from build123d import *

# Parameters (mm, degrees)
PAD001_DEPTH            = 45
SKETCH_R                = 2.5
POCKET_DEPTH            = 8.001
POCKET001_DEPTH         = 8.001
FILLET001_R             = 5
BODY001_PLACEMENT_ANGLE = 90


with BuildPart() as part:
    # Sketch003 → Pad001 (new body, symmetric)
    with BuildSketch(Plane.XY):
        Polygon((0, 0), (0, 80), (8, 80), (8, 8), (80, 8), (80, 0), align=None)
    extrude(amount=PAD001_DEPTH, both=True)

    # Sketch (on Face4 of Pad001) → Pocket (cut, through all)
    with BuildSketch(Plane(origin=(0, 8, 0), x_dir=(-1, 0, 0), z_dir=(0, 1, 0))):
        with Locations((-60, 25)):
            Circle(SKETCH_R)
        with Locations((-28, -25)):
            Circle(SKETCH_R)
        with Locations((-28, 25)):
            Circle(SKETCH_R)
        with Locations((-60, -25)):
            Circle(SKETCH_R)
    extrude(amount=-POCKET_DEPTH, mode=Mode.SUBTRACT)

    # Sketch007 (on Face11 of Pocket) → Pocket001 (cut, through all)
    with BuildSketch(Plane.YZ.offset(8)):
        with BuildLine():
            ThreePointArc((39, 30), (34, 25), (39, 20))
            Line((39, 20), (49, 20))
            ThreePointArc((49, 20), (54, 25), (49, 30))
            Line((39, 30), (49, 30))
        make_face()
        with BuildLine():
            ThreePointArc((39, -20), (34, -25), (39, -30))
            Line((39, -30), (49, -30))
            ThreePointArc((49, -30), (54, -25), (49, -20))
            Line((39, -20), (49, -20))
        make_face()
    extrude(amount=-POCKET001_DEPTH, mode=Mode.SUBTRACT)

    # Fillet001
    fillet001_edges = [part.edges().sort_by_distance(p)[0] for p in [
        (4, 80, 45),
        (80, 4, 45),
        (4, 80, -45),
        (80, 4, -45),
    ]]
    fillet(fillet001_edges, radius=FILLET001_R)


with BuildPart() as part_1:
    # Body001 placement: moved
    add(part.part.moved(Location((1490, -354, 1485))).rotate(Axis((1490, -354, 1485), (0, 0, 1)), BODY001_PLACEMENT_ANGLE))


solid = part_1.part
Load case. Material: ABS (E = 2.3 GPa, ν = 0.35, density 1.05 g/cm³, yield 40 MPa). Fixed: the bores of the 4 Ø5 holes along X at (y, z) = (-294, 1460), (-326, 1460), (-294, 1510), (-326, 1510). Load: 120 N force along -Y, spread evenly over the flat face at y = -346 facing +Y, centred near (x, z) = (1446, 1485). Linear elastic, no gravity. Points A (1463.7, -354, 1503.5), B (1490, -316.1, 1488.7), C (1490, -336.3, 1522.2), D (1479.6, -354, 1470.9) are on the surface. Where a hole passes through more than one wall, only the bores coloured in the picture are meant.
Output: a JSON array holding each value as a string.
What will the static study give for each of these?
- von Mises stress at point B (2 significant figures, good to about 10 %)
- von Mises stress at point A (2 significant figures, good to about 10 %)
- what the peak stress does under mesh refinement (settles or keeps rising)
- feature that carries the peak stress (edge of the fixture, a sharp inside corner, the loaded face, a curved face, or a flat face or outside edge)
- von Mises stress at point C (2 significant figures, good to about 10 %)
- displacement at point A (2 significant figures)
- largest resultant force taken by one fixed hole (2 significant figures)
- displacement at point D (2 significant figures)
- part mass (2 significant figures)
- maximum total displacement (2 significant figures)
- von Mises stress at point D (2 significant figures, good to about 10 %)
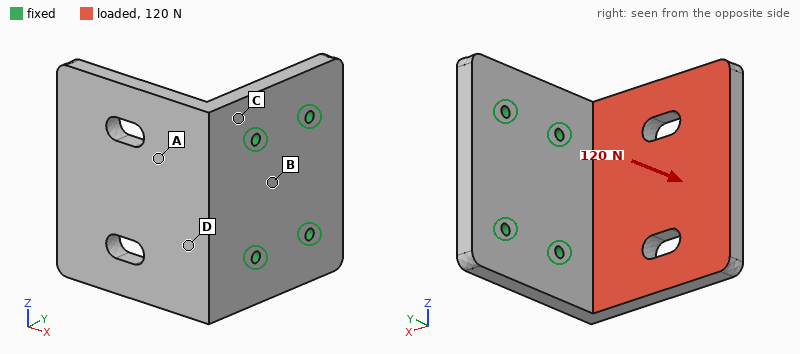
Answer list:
["1.3 MPa", "2.2 MPa", "keeps rising", "edge of the fixture", "4.4 MPa", "0.46 mm", "59 N", "0.26 mm", "110 g", "1.7 mm", "3.8 MPa"]
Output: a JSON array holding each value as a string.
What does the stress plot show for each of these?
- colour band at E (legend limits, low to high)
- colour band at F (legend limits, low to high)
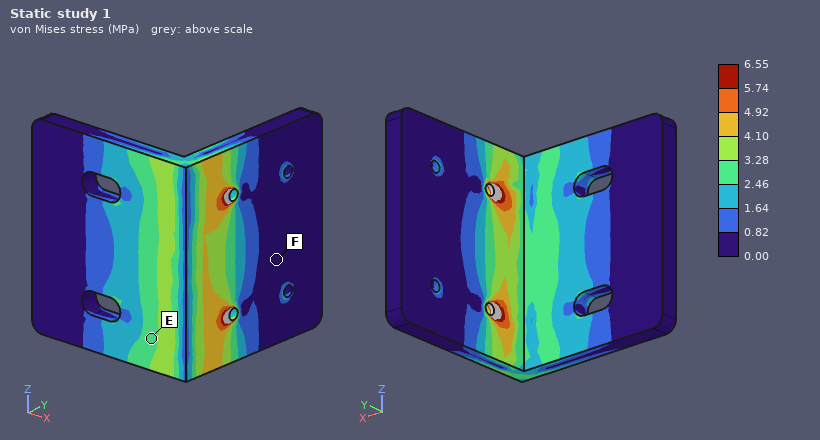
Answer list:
["2.46 to 3.28 MPa", "0.00 to 0.82 MPa"]
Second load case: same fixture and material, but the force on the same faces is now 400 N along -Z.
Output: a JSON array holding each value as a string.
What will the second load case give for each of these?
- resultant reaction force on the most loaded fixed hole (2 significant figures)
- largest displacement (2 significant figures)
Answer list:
["390 N", "0.99 mm"]
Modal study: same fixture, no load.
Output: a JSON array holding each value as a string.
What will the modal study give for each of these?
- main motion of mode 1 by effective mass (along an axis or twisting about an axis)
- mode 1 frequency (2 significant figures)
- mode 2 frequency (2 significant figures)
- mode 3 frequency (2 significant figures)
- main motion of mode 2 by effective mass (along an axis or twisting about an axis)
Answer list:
["along Y", "230 Hz", "500 Hz", "720 Hz", "along Z"]
